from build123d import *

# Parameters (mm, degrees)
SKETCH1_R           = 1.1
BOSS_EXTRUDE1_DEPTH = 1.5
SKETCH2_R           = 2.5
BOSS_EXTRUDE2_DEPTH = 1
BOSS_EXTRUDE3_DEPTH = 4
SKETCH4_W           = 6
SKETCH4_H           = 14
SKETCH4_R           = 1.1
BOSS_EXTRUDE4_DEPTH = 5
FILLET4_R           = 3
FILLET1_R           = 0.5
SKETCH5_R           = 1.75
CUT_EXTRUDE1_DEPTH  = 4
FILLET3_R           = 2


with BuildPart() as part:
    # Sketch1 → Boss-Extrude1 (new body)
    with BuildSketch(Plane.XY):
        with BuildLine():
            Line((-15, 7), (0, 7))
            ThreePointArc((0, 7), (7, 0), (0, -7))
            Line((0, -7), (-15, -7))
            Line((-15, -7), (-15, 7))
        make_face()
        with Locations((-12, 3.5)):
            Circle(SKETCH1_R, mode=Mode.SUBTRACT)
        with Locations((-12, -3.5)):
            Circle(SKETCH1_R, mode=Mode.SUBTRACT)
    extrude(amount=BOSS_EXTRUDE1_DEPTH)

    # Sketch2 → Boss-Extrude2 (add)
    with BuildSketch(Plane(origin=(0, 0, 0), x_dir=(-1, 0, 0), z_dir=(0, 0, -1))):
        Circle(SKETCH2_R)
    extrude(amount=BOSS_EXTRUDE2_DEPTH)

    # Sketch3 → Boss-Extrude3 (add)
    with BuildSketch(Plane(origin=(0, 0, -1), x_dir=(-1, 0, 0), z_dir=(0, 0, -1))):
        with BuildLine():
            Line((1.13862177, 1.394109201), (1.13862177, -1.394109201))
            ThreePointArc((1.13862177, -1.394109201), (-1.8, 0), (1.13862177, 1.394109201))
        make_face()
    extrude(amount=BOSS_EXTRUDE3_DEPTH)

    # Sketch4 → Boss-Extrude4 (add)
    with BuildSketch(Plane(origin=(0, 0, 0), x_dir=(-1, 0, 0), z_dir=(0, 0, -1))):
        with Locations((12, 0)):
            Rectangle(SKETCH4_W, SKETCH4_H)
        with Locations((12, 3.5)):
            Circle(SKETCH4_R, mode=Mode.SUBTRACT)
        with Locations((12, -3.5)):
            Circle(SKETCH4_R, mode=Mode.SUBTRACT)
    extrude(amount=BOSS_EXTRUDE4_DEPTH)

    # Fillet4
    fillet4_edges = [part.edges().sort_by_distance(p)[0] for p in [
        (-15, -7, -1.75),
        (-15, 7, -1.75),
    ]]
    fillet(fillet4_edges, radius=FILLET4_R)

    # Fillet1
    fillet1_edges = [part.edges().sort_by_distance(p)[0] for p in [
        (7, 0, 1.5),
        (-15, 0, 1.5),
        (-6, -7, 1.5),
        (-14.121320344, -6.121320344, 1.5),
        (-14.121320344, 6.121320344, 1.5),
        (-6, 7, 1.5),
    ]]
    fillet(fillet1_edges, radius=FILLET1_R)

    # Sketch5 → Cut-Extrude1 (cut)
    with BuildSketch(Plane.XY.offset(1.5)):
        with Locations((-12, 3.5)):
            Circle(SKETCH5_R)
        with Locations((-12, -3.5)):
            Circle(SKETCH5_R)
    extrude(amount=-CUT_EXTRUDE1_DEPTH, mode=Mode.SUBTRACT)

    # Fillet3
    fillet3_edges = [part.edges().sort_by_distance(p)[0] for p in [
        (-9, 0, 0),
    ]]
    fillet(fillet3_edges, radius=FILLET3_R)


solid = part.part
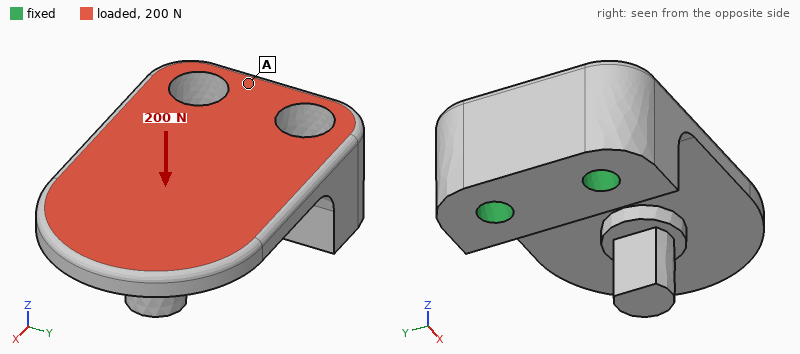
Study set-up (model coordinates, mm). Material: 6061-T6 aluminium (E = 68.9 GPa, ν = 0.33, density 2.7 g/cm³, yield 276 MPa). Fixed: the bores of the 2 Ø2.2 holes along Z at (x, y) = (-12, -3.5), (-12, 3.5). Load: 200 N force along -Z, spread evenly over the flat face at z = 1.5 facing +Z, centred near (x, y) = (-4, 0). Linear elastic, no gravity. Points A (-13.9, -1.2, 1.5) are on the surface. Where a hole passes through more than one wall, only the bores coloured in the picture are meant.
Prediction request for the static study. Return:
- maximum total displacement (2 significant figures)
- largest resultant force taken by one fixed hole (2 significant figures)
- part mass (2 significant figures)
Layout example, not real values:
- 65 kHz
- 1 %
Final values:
- 0.24 mm
- 110 N
- 2.1 g
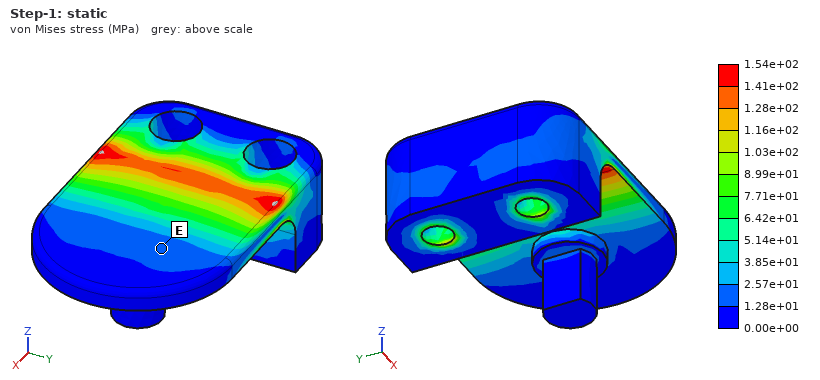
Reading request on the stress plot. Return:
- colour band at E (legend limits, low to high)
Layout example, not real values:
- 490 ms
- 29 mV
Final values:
- 1.28e+01 to 2.57e+01 MPa
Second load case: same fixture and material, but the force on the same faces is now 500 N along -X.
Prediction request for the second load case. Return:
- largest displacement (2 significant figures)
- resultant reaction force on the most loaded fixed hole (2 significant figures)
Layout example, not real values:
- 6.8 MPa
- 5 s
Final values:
- 0.12 mm
- 250 N
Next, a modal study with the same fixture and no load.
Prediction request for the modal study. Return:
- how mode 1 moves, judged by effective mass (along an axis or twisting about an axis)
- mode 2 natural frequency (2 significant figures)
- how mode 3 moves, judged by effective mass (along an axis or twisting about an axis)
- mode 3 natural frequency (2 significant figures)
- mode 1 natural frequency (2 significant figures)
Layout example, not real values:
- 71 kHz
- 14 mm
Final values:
- along Z
- 14 kHz
- along Y
- 20 kHz
- 5200 Hz
